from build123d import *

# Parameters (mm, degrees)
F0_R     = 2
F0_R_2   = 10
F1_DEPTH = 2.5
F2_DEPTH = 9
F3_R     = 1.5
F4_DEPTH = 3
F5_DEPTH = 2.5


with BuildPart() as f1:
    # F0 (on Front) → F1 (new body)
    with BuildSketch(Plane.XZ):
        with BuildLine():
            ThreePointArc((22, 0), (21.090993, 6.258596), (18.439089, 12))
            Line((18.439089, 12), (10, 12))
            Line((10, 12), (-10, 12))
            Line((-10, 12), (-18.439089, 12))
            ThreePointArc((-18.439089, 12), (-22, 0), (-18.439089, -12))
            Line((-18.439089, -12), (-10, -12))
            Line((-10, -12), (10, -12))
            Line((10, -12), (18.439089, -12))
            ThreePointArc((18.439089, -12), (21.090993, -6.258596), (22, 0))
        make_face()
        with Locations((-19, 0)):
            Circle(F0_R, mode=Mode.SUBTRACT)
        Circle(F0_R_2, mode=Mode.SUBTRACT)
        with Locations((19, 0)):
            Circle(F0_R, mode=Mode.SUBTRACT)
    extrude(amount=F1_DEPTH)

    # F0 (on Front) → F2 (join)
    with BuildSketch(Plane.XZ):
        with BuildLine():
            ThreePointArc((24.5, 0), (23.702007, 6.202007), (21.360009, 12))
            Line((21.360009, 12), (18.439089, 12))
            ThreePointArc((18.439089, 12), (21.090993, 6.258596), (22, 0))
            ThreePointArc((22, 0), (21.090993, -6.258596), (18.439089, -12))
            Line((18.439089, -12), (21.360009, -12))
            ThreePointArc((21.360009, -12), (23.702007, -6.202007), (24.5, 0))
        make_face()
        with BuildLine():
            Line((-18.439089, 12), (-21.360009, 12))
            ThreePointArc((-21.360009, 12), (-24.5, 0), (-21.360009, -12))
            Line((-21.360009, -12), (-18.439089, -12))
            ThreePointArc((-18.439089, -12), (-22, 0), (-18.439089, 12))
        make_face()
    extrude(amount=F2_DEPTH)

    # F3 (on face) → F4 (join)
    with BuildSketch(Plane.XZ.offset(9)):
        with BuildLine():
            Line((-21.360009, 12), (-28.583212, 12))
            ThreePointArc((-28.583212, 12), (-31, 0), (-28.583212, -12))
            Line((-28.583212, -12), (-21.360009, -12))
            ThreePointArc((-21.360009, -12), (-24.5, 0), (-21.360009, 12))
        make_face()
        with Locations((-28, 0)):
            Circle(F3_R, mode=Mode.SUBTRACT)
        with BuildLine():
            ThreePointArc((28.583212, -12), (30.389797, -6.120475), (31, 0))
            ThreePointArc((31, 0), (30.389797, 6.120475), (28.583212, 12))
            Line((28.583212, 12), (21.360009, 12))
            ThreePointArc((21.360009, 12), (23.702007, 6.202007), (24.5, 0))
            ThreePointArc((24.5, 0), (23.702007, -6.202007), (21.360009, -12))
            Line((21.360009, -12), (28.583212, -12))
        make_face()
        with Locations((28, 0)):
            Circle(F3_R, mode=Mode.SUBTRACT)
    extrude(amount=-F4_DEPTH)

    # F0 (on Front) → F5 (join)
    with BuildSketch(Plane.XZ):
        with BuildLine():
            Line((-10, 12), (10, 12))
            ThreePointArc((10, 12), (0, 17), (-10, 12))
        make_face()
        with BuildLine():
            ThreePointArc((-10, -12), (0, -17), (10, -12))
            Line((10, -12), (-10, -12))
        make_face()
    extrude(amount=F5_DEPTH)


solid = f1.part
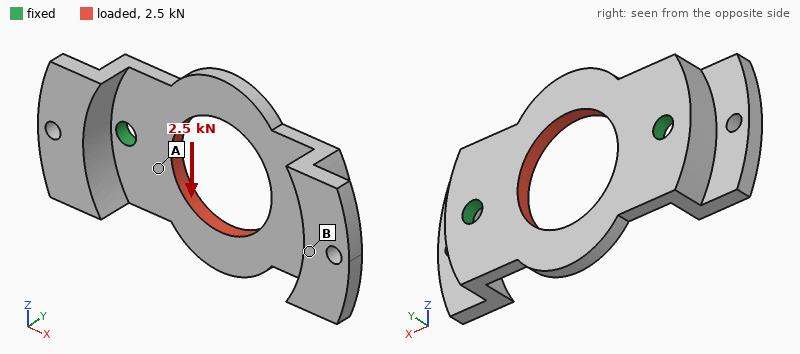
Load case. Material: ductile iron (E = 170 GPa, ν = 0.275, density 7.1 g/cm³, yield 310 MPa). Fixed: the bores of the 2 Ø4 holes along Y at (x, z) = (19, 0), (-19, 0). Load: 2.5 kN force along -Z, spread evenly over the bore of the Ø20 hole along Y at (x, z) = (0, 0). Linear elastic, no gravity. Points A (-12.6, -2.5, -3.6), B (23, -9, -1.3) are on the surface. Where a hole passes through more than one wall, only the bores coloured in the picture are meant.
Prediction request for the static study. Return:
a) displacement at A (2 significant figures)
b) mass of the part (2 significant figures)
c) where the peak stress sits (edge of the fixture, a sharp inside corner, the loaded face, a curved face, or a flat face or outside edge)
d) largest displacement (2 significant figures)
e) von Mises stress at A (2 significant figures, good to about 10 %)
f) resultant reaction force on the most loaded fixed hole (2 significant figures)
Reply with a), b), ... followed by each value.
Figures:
a) 3.6 µm
b) 29 g
c) edge of the fixture
d) 7.3 µm
e) 45 MPa
f) 1.3 kN
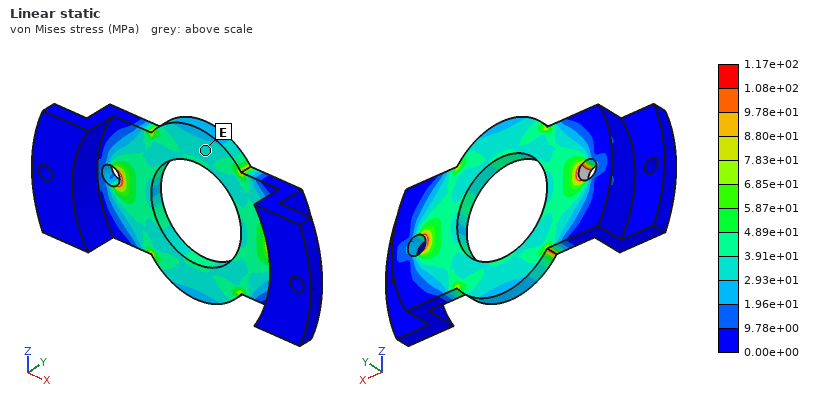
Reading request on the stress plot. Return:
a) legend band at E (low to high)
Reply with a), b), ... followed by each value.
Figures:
a) 2.93e+01 to 3.91e+01 MPa
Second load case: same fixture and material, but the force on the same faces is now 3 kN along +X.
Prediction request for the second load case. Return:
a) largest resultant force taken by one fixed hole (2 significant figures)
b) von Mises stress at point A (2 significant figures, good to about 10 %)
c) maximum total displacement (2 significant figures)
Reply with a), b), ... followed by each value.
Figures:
a) 1.5 kN
b) 45 MPa
c) 5.6 µm
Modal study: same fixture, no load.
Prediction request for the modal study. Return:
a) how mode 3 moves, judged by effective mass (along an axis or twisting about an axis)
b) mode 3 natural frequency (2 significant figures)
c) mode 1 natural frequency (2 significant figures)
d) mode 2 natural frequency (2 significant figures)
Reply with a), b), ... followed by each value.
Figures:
a) along X
b) 9000 Hz
c) 6500 Hz
d) 6600 Hz
